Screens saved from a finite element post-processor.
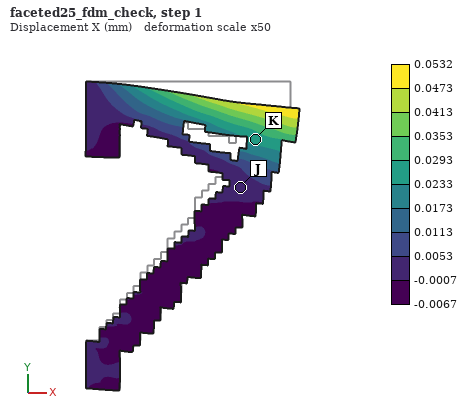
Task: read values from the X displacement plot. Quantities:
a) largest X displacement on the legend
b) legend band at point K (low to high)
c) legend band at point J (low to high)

0.0532 mm
0.0233 to 0.0293 mm
-0.0007 to 0.0053 mm
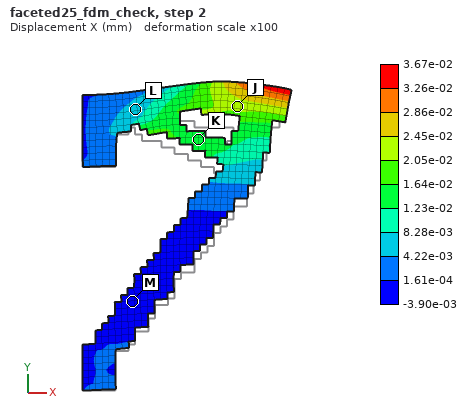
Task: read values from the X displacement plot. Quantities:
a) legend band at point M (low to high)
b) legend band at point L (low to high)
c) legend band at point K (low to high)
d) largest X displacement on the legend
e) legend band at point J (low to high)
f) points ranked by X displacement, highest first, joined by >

-3.90e-03 to 1.61e-04 mm
4.22e-03 to 8.28e-03 mm
1.23e-02 to 1.64e-02 mm
3.67e-02 mm
2.05e-02 to 2.45e-02 mm
J > K > L > M
